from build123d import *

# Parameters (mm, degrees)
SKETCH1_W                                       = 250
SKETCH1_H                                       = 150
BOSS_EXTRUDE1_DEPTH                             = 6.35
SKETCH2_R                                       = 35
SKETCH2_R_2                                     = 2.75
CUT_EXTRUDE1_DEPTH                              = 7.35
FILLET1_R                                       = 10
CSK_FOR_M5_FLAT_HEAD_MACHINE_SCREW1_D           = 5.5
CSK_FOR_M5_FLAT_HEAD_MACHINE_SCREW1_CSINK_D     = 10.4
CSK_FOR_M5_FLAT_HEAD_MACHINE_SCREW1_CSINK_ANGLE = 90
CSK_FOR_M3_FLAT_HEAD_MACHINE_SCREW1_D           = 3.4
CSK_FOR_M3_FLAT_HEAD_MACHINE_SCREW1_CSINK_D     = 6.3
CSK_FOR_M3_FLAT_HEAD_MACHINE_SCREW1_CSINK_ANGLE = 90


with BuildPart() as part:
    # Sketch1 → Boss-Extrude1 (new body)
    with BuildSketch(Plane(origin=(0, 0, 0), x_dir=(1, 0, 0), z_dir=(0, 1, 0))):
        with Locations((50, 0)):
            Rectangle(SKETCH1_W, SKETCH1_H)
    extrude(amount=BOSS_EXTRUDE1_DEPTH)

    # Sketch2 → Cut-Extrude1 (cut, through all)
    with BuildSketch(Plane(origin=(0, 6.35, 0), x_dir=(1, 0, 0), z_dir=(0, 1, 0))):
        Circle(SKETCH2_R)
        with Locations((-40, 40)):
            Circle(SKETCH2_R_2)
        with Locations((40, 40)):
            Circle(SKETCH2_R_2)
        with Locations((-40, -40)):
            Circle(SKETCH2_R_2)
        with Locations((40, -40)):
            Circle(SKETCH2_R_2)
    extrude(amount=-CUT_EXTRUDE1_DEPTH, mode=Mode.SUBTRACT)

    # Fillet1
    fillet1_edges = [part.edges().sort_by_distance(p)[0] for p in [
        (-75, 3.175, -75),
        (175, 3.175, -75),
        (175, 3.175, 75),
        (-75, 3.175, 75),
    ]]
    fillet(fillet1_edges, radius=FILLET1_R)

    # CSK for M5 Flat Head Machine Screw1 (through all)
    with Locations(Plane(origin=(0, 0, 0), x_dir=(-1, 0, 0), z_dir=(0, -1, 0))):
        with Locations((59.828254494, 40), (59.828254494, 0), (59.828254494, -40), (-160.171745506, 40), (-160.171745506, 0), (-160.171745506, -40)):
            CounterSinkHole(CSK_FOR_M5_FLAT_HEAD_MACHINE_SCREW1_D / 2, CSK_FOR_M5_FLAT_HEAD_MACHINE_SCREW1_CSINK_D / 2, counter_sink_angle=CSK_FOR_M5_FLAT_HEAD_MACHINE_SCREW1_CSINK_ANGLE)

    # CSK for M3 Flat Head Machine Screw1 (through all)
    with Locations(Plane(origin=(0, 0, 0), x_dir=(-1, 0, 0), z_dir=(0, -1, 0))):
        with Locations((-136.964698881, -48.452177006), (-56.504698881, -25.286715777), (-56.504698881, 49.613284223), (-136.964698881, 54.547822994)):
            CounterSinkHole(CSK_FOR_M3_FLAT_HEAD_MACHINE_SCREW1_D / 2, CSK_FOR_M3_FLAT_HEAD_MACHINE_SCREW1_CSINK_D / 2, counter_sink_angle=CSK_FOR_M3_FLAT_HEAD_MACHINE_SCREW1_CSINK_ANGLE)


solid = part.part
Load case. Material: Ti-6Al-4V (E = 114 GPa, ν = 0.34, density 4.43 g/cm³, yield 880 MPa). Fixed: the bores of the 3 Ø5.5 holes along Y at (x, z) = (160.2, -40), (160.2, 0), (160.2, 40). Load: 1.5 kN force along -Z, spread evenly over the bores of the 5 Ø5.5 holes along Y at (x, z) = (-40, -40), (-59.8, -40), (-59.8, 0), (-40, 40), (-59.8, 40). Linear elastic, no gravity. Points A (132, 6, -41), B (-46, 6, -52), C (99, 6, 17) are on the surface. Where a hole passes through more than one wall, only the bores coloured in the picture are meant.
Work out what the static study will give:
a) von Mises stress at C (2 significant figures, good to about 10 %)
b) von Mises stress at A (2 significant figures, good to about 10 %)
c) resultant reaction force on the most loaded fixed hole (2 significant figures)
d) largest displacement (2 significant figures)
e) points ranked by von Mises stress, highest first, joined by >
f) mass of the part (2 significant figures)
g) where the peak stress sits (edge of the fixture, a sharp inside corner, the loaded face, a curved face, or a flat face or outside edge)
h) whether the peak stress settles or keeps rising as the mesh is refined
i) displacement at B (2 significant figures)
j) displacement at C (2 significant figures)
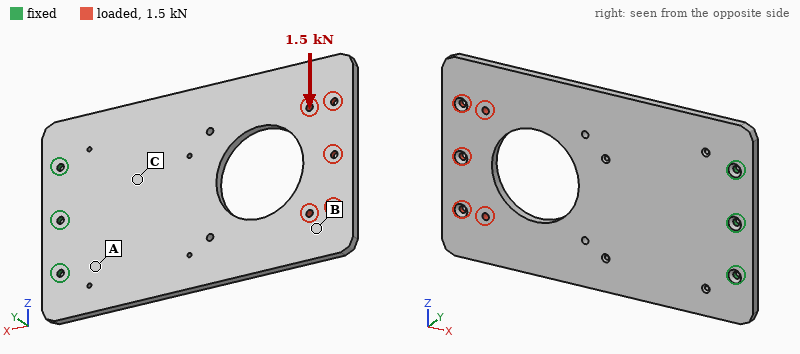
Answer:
7.3 MPa
13 MPa
3.8 kN
93 µm
A > C > B
930 g
edge of the fixture
keeps rising
77 µm
15 µm
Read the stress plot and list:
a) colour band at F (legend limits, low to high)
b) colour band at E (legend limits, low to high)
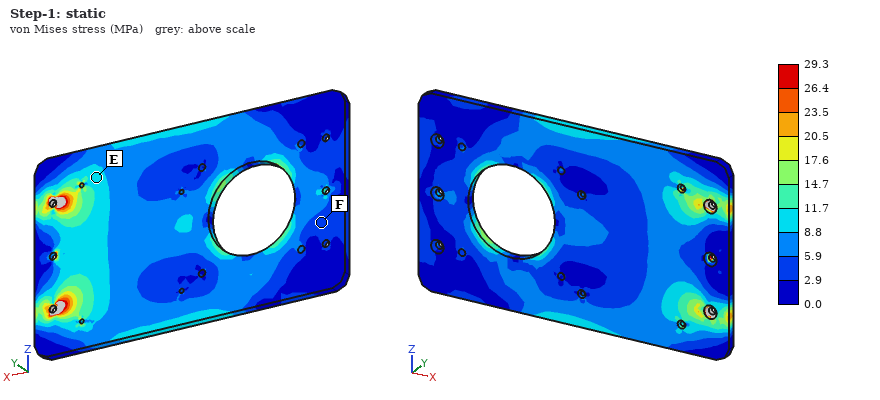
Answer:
2.9 to 5.9 MPa
8.8 to 11.7 MPa
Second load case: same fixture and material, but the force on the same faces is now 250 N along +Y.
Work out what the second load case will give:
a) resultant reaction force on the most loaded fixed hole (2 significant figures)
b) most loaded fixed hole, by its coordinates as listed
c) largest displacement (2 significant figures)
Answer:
300 N
(160.2, 0)
3.0 mm
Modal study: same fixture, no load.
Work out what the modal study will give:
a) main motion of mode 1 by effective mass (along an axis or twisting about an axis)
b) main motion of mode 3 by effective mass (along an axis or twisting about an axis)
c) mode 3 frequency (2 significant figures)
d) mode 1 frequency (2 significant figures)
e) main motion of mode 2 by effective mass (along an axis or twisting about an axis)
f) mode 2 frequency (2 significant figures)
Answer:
along Y
along Y
510 Hz
95 Hz
twisting about X
300 Hz
